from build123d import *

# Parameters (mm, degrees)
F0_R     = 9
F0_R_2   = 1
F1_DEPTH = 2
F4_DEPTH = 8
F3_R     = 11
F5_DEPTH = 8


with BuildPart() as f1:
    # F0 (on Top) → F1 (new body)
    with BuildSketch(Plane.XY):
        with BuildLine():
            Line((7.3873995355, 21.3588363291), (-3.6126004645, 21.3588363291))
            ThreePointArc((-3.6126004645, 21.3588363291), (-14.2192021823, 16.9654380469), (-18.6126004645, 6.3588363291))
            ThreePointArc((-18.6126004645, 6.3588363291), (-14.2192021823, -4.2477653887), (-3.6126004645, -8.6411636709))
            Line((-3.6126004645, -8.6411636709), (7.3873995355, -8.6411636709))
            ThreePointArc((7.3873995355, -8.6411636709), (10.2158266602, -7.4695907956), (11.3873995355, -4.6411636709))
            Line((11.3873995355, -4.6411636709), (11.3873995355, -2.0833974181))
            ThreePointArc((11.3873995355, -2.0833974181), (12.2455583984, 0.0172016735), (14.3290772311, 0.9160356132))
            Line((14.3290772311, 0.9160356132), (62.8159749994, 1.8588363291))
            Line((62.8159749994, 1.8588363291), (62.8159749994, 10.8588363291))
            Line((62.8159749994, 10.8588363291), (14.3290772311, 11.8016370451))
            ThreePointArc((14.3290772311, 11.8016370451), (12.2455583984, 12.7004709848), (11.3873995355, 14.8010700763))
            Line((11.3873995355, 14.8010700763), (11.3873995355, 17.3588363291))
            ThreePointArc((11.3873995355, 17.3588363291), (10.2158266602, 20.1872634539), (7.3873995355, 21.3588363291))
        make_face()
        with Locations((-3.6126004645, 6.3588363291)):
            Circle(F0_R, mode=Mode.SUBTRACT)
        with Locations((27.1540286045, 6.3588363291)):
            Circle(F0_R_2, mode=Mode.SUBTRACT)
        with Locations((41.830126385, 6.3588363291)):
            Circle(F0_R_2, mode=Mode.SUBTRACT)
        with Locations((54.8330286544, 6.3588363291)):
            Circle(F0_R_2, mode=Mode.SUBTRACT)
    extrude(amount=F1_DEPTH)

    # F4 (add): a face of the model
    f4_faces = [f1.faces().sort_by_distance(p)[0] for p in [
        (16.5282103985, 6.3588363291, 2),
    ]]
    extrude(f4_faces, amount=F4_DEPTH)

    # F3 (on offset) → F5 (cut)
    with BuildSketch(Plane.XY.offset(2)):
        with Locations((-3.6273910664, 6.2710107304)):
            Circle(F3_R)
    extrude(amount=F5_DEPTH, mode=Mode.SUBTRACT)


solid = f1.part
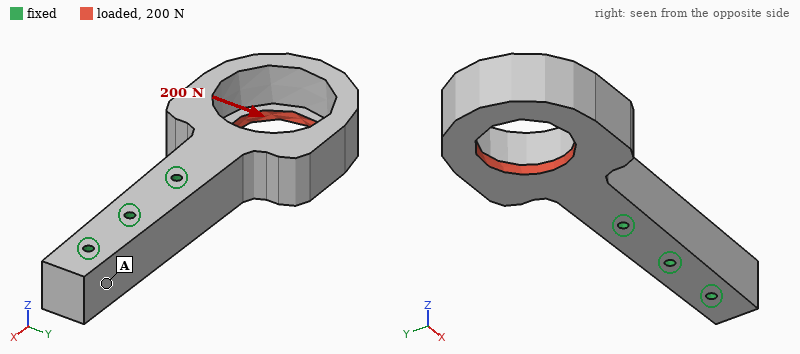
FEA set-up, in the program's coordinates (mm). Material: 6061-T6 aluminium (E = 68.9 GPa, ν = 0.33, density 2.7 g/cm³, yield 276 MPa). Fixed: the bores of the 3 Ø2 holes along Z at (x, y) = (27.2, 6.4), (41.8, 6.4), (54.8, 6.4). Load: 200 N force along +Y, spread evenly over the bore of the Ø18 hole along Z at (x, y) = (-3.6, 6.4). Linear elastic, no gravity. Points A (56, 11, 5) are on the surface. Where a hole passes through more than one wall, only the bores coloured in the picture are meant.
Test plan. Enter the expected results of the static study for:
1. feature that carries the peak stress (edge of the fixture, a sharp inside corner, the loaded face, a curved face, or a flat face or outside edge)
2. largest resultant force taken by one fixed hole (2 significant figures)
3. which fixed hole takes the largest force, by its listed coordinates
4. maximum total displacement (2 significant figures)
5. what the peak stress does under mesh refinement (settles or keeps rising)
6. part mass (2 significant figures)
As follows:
edge of the fixture
520 N
(27.2, 6.4)
81 µm
keeps rising
26 g
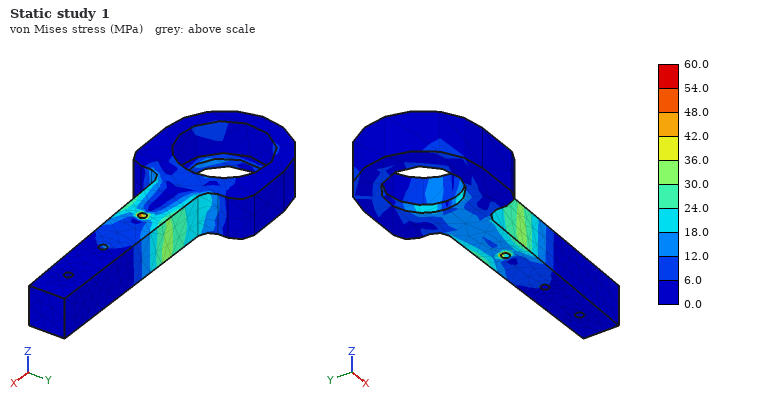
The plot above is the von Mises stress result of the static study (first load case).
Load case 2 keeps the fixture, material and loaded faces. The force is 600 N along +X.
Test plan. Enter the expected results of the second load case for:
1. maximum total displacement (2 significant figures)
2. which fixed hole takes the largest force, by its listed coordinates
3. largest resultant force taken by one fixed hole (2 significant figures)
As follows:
43 µm
(27.2, 6.4)
520 N
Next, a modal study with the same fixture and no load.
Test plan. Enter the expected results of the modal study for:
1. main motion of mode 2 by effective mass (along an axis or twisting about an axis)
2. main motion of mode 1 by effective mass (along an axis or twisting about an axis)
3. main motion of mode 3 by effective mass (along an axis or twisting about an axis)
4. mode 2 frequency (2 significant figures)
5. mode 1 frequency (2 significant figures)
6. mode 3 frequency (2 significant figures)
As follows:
along Z
along Y
twisting about X
3200 Hz
2800 Hz
6300 Hz
